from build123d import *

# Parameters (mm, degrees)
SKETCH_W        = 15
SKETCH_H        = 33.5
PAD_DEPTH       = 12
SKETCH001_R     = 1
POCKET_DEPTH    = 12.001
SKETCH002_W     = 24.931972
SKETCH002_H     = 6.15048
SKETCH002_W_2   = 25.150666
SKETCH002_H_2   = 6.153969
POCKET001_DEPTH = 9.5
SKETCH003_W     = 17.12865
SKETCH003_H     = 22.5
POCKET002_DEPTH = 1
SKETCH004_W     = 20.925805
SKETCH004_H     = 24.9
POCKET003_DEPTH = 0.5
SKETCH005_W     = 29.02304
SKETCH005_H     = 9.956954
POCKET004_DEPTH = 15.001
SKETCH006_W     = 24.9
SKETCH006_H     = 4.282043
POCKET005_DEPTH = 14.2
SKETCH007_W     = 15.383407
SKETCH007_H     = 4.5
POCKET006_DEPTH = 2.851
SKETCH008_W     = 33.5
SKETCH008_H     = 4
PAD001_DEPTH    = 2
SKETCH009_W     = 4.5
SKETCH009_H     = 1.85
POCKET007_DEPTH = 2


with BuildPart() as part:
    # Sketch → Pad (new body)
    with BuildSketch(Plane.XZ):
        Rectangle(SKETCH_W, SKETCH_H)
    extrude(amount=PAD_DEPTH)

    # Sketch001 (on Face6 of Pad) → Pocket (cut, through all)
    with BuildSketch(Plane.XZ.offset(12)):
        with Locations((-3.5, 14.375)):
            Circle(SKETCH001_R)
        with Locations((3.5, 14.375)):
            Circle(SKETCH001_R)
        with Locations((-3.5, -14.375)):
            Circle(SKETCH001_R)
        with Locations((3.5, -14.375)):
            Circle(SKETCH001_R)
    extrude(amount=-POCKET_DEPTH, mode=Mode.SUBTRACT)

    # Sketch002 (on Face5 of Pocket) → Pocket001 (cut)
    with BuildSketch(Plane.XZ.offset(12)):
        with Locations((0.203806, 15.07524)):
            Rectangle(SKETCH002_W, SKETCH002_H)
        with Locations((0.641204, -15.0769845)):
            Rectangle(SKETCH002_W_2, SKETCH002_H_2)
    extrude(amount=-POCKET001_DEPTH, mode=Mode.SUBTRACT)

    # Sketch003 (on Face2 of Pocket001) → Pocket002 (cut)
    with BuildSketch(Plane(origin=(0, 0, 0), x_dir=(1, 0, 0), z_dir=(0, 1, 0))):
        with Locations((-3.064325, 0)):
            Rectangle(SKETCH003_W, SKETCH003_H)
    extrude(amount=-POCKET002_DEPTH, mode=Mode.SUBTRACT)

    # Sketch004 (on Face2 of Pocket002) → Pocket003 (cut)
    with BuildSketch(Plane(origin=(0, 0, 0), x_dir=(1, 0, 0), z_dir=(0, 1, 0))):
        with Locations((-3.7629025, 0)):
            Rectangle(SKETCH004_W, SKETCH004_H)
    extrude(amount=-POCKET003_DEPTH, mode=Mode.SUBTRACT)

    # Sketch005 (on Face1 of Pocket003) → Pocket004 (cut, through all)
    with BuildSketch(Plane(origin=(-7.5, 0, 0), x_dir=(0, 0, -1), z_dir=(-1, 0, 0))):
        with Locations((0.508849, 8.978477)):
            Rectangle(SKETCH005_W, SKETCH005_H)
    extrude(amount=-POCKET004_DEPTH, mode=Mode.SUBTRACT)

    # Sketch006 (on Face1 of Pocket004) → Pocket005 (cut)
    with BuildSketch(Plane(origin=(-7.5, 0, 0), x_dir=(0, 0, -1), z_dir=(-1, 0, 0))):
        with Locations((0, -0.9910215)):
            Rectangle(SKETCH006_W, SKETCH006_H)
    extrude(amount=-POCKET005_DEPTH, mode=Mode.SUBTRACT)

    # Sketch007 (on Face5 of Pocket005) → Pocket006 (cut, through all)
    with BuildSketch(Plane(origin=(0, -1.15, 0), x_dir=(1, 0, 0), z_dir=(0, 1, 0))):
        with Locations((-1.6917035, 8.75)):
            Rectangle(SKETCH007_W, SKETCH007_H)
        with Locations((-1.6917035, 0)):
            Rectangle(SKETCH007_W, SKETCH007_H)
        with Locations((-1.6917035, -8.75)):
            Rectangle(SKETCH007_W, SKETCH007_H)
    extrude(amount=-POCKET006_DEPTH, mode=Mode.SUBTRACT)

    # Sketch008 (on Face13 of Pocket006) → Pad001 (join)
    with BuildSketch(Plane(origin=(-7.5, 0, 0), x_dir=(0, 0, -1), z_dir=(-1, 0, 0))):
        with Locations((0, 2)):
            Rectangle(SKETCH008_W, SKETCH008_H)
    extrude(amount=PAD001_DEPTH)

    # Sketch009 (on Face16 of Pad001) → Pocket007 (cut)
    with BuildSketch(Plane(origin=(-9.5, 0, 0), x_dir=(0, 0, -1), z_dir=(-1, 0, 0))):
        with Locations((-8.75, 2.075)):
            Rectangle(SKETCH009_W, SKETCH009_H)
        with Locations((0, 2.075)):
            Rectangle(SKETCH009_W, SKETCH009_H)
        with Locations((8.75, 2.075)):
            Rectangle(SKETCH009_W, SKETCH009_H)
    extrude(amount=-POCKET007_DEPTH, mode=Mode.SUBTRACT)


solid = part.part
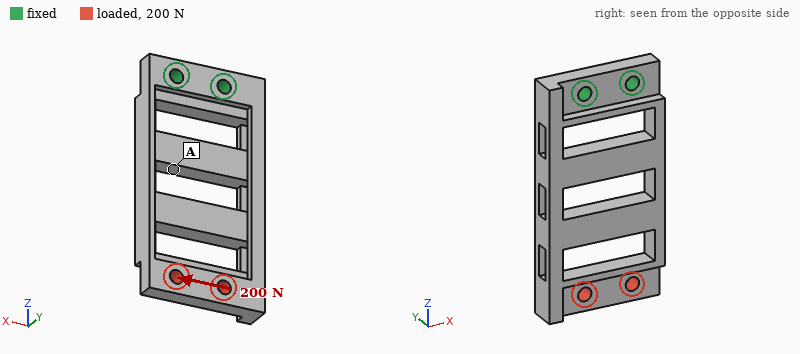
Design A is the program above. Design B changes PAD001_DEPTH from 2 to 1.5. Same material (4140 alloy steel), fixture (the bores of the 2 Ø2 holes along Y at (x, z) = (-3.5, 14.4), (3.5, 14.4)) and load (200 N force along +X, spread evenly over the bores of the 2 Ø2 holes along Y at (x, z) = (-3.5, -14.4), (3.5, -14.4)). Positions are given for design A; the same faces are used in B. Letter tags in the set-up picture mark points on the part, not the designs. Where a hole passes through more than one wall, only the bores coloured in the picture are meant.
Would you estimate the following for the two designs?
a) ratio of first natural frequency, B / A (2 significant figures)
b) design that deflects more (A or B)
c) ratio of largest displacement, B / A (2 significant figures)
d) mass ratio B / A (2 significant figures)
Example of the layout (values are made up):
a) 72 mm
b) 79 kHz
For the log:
a) 0.97
b) B
c) 1.2
d) 0.95
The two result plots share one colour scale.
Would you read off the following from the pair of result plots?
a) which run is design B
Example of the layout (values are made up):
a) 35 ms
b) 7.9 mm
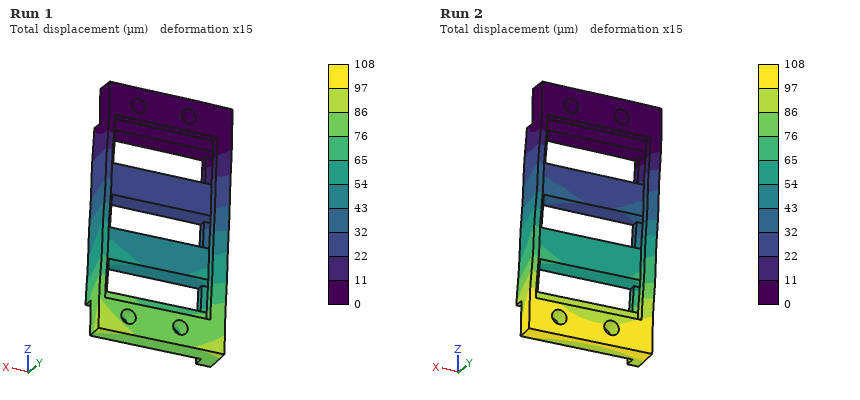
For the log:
a) Run 2
